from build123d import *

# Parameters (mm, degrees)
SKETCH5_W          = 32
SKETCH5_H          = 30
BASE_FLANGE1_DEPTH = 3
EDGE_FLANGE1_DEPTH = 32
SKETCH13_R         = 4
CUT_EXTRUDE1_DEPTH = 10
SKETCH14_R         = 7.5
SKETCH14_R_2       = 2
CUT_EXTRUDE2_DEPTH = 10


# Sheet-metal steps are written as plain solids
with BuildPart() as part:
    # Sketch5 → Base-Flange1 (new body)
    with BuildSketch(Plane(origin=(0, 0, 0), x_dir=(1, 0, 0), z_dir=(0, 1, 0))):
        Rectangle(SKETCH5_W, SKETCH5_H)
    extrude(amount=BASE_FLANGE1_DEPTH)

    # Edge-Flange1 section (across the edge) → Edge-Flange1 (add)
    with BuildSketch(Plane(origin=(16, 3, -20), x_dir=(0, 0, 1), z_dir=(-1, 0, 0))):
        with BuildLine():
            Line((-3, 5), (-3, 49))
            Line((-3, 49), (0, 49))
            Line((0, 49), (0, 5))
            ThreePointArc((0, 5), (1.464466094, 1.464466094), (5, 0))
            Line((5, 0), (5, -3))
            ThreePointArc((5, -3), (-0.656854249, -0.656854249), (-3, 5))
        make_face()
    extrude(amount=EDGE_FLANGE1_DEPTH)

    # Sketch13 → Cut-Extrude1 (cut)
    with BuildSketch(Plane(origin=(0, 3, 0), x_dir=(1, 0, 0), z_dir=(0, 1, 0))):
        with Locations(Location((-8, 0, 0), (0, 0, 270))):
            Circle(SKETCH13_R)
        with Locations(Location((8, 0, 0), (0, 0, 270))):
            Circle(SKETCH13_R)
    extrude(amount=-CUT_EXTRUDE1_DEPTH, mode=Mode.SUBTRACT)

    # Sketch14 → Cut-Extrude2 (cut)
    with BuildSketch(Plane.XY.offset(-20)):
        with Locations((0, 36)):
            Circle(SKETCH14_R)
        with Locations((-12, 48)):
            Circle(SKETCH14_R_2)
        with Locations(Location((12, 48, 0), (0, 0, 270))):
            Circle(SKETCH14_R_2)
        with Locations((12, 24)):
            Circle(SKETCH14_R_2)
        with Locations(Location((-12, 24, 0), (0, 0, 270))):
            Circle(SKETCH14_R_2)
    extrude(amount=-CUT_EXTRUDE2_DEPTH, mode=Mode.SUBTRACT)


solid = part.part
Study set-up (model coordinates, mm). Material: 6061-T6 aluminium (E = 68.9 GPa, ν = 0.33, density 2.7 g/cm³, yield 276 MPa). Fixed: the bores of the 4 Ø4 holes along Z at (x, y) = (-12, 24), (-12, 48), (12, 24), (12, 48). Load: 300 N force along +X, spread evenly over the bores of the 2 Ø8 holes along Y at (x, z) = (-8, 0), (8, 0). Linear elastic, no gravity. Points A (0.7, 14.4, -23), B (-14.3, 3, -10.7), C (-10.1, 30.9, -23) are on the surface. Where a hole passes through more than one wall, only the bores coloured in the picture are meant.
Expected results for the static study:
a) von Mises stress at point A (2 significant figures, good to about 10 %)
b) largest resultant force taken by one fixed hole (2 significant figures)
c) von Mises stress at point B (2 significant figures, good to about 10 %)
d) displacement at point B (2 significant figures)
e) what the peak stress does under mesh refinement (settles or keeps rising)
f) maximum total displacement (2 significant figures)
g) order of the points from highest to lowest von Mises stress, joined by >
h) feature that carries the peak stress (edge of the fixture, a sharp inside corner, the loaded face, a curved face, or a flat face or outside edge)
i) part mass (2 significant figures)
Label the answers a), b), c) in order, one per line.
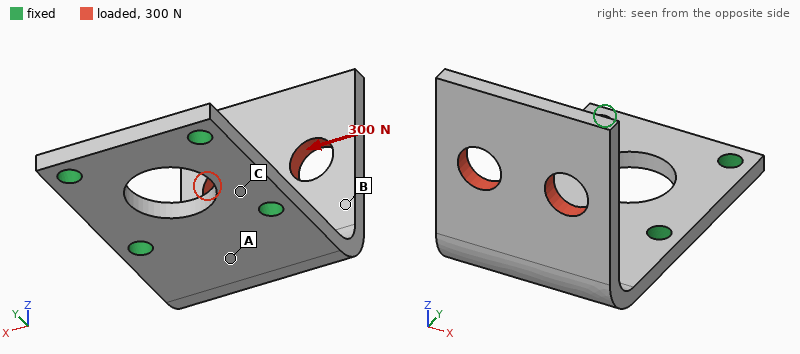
a) 59 MPa
b) 400 N
c) 34 MPa
d) 0.17 mm
e) keeps rising
f) 0.39 mm
g) A > B > C
h) edge of the fixture
i) 19 g
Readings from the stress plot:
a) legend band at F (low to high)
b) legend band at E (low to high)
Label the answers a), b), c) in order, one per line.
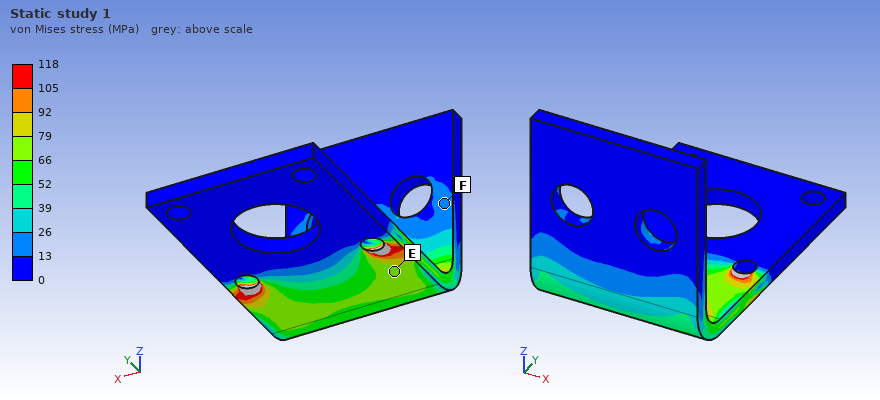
a) 13 to 26 MPa
b) 66 to 79 MPa
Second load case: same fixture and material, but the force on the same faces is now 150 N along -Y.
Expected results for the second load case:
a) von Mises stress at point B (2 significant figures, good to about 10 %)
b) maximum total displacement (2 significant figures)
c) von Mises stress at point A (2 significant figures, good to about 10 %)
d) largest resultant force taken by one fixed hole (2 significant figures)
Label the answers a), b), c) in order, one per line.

a) 31 MPa
b) 0.66 mm
c) 55 MPa
d) 77 N
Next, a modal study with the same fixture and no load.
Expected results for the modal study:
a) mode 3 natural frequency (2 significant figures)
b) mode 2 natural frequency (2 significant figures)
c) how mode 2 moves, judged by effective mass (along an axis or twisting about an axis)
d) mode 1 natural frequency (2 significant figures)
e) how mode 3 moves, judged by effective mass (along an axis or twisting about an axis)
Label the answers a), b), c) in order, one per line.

a) 3100 Hz
b) 1900 Hz
c) along X
d) 1000 Hz
e) along Z
